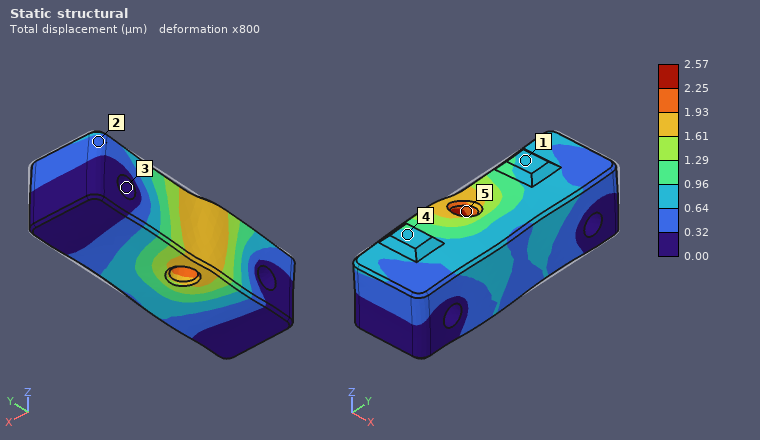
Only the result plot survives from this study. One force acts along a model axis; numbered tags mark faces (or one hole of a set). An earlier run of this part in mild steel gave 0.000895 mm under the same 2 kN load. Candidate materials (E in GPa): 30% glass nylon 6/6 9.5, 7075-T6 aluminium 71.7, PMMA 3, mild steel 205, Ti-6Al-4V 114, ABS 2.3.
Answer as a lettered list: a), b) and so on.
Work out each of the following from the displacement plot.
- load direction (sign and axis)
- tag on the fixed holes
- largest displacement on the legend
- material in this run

a) -Y
b) 3
c) 2.57 µm
d) 7075-T6 aluminium
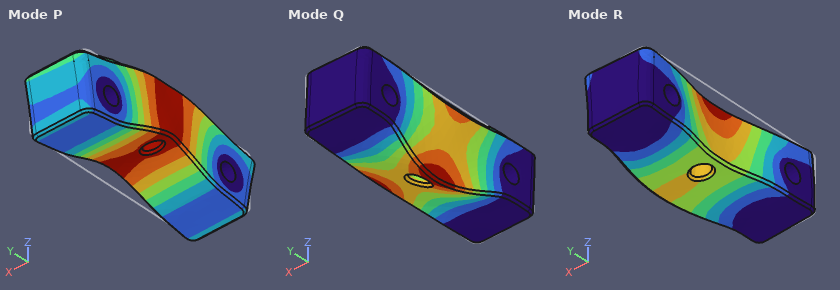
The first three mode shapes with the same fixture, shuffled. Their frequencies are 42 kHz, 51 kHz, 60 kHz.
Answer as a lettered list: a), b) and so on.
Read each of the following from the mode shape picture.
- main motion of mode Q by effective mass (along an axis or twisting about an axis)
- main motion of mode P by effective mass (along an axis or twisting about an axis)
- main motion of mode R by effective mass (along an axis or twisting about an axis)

a) twisting about Y
b) along Z
c) along X
